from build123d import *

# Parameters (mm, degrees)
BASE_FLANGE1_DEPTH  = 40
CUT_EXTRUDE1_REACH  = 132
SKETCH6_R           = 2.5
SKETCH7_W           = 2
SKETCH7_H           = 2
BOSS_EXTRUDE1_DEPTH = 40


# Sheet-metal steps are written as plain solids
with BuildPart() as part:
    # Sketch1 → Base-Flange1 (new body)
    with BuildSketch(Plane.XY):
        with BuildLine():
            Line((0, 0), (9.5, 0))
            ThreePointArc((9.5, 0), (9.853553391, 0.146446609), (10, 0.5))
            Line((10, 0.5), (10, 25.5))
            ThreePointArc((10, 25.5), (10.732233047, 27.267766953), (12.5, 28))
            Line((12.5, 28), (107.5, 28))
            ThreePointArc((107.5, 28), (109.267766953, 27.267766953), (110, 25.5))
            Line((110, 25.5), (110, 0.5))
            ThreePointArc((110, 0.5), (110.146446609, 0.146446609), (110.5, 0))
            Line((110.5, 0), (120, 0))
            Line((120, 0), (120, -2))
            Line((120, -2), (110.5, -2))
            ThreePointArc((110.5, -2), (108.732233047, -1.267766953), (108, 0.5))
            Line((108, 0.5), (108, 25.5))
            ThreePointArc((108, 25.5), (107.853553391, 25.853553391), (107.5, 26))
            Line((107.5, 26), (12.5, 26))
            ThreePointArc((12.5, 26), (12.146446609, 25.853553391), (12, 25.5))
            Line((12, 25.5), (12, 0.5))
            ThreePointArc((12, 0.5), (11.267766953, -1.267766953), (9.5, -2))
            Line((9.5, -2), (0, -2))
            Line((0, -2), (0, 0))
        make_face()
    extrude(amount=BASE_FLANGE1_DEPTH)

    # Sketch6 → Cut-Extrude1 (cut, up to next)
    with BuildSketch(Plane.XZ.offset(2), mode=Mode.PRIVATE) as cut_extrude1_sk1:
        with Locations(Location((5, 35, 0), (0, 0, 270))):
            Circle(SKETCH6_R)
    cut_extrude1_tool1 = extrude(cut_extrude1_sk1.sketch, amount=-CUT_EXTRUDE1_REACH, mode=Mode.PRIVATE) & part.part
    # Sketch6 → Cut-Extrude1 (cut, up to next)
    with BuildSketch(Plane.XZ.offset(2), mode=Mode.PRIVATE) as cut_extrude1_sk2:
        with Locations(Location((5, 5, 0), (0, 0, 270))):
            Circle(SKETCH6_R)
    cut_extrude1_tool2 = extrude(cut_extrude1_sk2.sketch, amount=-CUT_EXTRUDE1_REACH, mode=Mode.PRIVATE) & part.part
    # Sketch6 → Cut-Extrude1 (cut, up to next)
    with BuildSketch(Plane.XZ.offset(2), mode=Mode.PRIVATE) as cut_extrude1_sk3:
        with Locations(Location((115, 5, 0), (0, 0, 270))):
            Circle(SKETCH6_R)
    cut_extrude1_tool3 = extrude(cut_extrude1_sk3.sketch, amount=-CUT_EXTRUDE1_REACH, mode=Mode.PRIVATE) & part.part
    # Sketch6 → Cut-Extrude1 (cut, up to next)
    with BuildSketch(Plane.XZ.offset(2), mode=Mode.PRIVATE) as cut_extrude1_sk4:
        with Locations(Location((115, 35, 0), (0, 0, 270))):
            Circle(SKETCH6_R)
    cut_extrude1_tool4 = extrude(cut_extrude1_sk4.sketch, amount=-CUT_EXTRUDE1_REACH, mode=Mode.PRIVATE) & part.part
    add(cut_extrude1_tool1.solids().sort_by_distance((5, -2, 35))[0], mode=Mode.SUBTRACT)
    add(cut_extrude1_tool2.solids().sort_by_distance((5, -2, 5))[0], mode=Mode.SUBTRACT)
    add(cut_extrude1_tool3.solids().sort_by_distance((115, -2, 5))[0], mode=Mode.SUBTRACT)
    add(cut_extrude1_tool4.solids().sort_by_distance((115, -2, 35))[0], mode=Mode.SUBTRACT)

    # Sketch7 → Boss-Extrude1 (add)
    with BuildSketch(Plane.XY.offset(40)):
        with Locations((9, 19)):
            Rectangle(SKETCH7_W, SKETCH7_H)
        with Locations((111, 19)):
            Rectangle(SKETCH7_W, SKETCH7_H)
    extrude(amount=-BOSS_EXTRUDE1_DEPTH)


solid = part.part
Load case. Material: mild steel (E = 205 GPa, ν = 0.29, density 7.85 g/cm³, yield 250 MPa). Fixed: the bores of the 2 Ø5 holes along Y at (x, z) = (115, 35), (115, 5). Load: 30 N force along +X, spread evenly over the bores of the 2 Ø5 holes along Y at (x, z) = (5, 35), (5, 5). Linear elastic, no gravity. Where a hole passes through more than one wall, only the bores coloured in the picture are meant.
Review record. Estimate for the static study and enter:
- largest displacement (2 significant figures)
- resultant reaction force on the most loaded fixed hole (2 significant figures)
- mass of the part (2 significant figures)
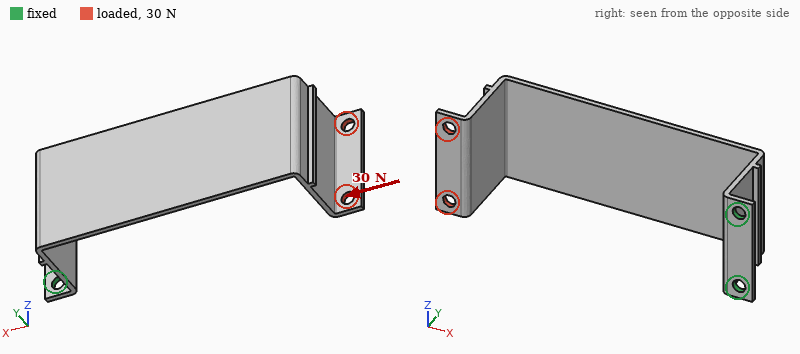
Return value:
1.2 mm
15 N
110 g
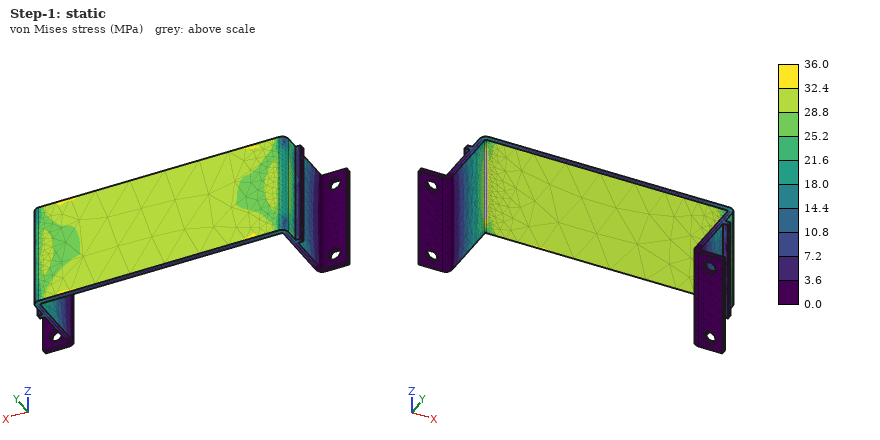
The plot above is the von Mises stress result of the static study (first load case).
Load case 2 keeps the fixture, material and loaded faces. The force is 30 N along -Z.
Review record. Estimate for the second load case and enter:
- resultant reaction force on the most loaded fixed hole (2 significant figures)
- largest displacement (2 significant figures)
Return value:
100 N
1.0 mm
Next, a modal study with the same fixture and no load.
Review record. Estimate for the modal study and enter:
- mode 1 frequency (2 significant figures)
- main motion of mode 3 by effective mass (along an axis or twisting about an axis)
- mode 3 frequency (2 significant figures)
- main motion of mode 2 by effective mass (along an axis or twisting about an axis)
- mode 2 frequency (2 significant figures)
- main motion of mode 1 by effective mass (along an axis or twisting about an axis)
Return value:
73 Hz
along X
360 Hz
along Z
160 Hz
along Y
